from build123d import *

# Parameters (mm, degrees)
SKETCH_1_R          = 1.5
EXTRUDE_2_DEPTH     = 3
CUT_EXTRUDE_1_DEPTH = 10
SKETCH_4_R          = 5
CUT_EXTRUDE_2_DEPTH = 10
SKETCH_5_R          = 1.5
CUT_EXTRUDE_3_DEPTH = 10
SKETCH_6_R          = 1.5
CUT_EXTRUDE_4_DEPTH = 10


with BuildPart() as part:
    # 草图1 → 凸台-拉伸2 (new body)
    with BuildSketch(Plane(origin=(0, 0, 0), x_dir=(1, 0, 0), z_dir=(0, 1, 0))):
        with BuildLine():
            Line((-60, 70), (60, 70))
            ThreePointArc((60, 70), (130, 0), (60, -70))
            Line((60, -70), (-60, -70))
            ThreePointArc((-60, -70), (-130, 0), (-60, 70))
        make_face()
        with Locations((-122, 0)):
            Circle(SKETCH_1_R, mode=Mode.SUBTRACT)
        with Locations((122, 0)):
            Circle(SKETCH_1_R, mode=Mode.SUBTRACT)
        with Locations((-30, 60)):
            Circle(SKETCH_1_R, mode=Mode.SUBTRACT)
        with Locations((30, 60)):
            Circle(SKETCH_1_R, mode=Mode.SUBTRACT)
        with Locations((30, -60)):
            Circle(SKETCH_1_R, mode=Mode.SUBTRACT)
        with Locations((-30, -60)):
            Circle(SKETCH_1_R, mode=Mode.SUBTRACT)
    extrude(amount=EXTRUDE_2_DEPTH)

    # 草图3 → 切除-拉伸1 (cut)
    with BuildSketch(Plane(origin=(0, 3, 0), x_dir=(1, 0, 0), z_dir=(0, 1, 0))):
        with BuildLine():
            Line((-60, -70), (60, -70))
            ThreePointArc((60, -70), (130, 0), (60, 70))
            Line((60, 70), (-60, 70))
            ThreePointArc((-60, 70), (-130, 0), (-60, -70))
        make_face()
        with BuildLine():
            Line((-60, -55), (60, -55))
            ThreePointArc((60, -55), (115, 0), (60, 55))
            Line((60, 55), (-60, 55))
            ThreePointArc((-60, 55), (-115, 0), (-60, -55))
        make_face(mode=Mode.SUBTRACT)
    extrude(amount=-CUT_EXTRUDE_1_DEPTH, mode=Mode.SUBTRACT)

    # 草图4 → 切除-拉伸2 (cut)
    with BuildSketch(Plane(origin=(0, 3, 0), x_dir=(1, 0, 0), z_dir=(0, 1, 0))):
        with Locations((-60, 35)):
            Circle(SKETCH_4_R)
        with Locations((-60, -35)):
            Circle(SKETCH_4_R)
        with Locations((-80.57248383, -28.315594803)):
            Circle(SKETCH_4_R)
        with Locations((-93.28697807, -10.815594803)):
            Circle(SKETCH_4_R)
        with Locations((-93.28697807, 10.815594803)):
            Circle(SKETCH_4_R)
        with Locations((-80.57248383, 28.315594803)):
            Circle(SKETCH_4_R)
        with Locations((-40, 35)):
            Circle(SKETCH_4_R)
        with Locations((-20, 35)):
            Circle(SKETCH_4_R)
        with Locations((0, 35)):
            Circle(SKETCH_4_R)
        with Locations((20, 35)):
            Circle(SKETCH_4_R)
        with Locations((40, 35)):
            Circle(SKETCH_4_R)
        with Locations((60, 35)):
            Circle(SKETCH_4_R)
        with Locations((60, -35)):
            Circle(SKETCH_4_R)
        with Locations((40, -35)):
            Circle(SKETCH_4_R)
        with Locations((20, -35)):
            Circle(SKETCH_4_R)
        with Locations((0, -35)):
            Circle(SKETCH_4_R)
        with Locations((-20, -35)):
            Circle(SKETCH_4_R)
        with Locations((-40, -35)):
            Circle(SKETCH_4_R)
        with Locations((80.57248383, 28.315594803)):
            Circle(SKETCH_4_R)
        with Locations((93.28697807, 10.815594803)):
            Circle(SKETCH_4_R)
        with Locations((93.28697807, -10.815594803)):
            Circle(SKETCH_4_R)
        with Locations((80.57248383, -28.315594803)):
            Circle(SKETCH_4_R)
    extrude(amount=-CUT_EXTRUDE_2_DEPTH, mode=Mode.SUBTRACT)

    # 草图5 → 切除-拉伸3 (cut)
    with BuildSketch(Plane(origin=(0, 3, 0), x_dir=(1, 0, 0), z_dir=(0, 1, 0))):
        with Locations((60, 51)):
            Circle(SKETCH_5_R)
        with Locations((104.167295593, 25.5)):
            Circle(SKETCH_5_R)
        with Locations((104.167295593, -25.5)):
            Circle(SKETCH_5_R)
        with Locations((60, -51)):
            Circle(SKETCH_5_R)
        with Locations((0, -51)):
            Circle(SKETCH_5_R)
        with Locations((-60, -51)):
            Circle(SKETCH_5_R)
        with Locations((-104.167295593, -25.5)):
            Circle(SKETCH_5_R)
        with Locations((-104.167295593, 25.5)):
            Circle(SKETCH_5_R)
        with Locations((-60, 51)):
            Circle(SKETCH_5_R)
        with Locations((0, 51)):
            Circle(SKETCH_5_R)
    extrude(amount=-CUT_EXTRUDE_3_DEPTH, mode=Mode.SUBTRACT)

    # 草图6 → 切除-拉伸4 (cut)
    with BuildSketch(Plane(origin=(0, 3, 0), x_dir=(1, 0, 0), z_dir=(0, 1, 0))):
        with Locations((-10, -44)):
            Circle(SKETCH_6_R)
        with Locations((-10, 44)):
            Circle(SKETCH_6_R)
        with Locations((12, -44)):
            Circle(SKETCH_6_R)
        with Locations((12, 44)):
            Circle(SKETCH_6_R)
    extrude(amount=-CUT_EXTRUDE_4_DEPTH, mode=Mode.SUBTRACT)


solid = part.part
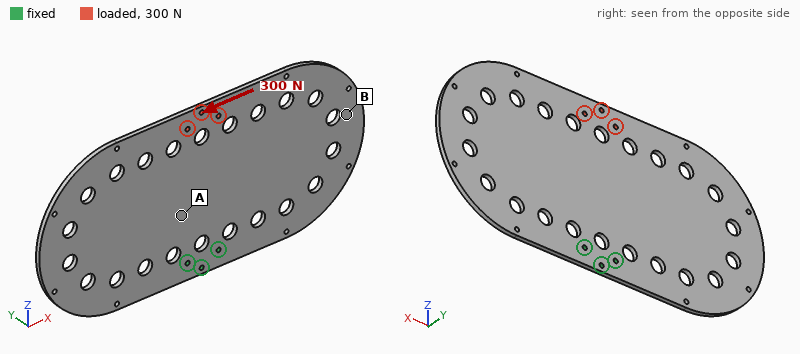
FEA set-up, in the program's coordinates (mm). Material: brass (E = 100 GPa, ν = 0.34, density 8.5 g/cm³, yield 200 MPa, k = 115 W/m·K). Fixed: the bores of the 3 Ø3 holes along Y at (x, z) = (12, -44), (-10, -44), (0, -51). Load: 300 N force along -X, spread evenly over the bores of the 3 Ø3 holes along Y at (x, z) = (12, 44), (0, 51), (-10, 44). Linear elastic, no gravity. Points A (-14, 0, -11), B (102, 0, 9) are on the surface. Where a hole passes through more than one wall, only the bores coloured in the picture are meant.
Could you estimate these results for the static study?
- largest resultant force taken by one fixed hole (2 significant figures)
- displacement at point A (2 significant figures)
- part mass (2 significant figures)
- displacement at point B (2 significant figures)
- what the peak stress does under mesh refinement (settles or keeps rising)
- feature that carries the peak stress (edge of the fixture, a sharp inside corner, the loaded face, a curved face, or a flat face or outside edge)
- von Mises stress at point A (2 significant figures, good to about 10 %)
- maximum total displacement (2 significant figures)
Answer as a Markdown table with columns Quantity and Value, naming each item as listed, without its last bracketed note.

| Quantity | Value |
|---|---|
| largest resultant force taken by one fixed hole | 1.1 kN |
| displacement at point A | 18 µm |
| part mass | 530 g |
| displacement at point B | 55 µm |
| what the peak stress does under mesh refinement | keeps rising |
| feature that carries the peak stress | edge of the fixture |
| von Mises stress at point A | 5.1 MPa |
| maximum total displacement | 63 µm |
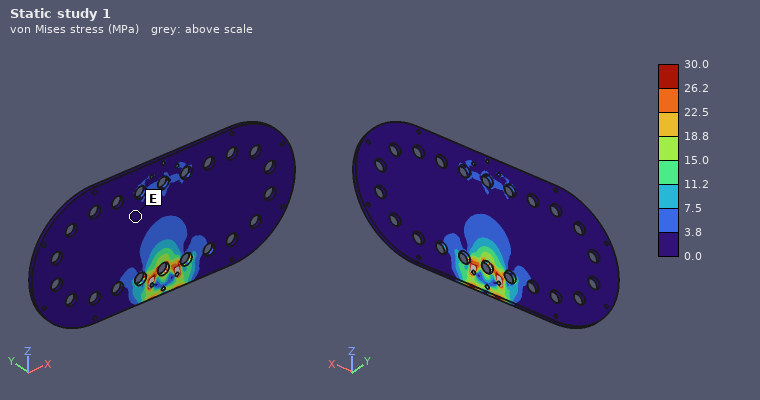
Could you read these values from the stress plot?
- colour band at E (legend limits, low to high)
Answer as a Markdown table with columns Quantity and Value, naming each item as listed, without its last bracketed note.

| Quantity | Value |
|---|---|
| colour band at E | 0.0 to 3.8 MPa |
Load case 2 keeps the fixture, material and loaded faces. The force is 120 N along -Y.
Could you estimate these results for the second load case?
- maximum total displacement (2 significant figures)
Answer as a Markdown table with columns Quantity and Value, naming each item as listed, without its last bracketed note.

| Quantity | Value |
|---|---|
| maximum total displacement | 2.0 mm |
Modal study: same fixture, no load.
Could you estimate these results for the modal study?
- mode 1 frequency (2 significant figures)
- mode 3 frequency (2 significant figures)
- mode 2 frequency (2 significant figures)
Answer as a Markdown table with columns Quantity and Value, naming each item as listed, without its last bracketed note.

| Quantity | Value |
|---|---|
| mode 1 frequency | 100 Hz |
| mode 3 frequency | 200 Hz |
| mode 2 frequency | 100 Hz |
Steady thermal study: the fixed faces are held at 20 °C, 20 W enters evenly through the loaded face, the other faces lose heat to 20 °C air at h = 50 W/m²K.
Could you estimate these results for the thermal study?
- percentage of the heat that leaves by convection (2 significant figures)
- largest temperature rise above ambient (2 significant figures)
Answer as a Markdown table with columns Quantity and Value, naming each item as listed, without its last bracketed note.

| Quantity | Value |
|---|---|
| percentage of the heat that leaves by convection | 85 % |
| largest temperature rise above ambient | 43 K |
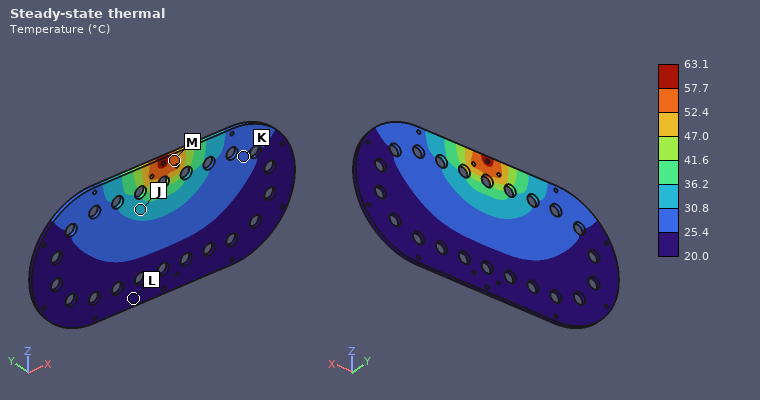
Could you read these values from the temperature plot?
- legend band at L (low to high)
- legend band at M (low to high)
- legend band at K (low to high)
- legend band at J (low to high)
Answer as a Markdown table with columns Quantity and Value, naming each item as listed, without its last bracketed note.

| Quantity | Value |
|---|---|
| legend band at L | 20.0 to 25.4 °C |
| legend band at M | 52.4 to 57.7 °C |
| legend band at K | 25.4 to 30.8 °C |
| legend band at J | 30.8 to 36.2 °C |
